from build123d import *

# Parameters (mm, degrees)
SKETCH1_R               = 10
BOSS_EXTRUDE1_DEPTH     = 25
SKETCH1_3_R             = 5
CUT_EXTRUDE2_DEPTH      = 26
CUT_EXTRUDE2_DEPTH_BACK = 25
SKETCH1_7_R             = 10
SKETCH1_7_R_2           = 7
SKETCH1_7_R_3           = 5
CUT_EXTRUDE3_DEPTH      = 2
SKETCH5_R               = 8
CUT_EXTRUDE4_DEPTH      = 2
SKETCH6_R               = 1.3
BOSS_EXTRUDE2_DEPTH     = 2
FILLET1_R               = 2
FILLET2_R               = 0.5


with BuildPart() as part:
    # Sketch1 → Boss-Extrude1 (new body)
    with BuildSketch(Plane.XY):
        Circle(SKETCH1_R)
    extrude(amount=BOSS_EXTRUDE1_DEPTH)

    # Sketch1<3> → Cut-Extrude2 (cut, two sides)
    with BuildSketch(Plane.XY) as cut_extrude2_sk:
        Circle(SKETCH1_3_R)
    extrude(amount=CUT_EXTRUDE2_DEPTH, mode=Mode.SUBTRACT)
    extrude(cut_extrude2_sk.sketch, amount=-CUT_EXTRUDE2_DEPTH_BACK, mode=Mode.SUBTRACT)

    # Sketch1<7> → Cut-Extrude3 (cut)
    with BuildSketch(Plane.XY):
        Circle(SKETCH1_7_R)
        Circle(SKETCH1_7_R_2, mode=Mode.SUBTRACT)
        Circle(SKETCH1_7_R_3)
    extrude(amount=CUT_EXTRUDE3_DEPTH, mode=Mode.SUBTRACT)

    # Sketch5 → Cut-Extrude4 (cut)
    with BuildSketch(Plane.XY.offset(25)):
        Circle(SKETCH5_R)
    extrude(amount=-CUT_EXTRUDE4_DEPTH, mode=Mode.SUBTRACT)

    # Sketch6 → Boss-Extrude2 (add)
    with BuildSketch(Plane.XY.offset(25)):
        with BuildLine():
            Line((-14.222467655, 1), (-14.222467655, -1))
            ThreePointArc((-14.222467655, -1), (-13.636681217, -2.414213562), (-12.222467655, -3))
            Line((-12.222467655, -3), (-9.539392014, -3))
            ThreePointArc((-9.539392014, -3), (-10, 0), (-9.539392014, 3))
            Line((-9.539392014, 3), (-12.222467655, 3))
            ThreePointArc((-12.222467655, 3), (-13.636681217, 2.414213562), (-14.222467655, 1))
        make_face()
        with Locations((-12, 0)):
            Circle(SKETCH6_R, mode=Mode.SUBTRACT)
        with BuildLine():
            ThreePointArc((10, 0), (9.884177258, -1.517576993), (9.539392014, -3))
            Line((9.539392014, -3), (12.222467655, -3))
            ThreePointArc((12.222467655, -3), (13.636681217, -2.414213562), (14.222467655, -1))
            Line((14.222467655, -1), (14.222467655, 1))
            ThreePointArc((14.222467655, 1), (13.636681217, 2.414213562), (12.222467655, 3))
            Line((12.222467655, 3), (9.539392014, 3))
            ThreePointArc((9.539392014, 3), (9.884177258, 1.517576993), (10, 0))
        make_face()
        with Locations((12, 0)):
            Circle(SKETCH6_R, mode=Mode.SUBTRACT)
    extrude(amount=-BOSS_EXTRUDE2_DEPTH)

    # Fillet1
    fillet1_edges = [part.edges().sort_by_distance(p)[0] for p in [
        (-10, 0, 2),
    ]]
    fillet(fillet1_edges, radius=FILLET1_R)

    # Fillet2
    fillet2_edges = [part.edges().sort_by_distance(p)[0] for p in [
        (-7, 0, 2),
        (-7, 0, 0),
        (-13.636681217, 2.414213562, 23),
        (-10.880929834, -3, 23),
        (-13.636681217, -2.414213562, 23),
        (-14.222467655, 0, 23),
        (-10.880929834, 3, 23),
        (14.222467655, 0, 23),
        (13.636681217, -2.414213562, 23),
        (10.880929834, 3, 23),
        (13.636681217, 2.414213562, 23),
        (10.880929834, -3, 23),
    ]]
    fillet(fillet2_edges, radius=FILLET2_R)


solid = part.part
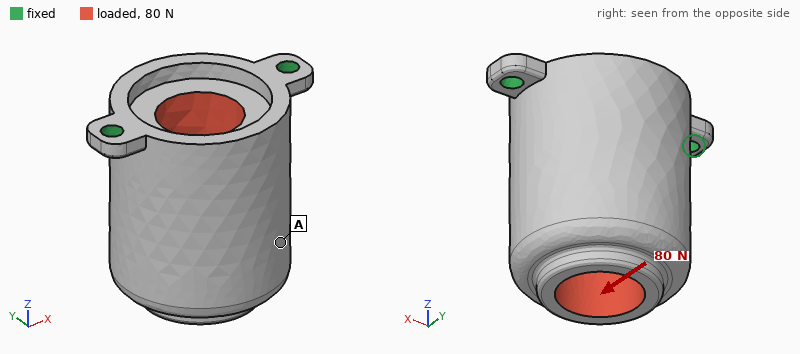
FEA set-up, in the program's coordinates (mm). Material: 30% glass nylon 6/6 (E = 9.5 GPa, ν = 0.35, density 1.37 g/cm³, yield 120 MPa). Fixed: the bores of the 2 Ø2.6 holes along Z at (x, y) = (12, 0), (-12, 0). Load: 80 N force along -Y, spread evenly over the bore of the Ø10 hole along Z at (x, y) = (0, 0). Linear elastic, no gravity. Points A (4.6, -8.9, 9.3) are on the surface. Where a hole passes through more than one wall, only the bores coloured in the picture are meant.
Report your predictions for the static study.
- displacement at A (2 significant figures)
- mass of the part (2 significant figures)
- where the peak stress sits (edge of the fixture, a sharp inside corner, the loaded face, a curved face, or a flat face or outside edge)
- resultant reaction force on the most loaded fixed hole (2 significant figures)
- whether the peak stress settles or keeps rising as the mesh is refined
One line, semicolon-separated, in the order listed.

0.30 mm; 7.3 g; edge of the fixture; 40 N; keeps rising
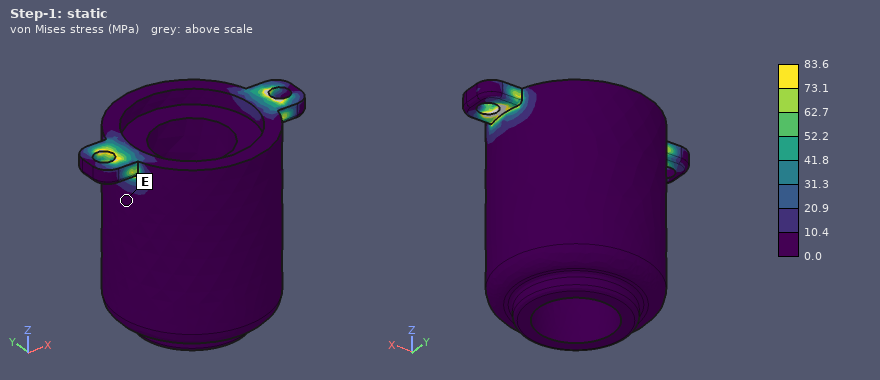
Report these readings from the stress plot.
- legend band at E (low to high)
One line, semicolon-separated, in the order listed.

0.0 to 10.4 MPa
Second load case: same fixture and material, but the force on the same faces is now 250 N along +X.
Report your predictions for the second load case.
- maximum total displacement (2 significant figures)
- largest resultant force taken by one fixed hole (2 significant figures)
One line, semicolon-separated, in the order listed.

45 µm; 200 N
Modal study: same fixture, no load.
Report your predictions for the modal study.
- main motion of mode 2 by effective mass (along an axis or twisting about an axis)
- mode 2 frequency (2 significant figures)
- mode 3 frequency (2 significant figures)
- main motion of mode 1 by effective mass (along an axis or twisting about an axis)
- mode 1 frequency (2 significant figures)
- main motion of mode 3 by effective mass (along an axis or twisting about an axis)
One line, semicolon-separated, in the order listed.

along X; 5500 Hz; 7800 Hz; along Y; 1000 Hz; along Z
